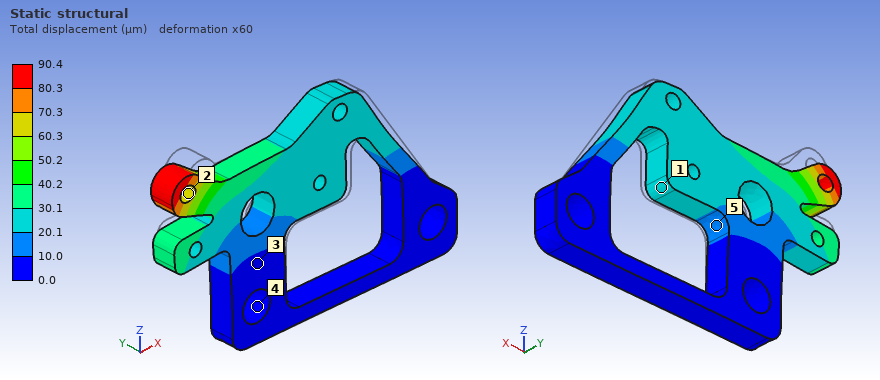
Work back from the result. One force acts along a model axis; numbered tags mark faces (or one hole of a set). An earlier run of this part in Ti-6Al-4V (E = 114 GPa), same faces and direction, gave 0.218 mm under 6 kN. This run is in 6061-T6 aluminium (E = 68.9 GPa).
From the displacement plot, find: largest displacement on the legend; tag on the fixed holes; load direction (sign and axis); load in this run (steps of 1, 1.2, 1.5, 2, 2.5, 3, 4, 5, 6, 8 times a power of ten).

90.4 µm
4
-X
1.5 kN
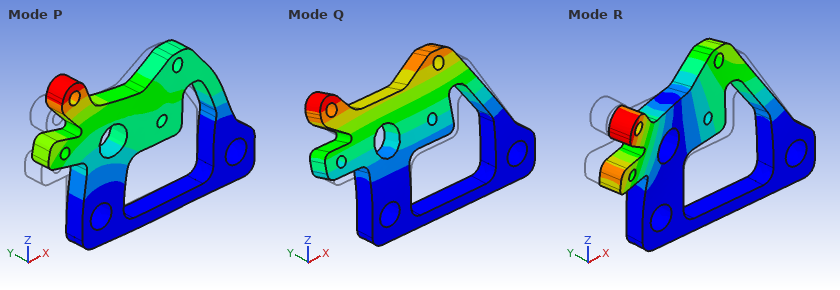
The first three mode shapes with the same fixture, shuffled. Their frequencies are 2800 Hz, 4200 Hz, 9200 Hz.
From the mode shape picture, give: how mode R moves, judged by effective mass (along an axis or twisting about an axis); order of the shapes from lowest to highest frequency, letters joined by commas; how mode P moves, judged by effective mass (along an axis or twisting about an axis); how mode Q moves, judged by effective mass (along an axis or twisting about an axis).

twisting about Z
Q, R, P
along X
along Y
